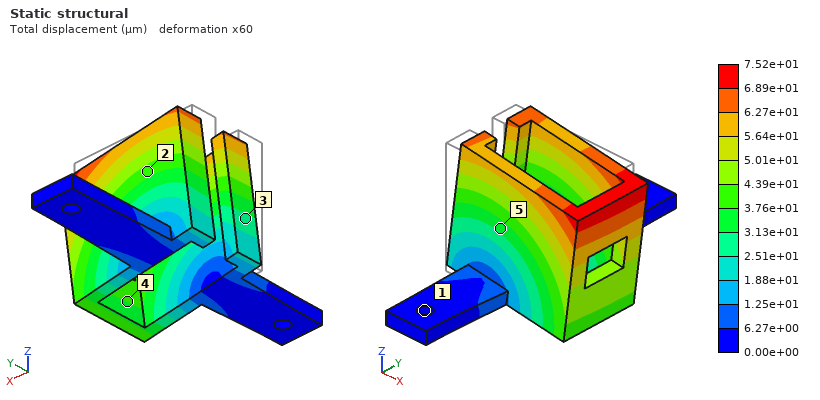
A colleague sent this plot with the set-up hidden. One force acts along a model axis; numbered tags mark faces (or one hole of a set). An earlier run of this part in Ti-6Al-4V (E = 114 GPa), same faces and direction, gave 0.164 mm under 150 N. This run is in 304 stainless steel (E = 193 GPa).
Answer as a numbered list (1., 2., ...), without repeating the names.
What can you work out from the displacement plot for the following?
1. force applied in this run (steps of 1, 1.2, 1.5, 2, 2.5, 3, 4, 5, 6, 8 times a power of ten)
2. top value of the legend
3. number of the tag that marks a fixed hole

1. 120 N
2. 7.52e+01 µm
3. 1
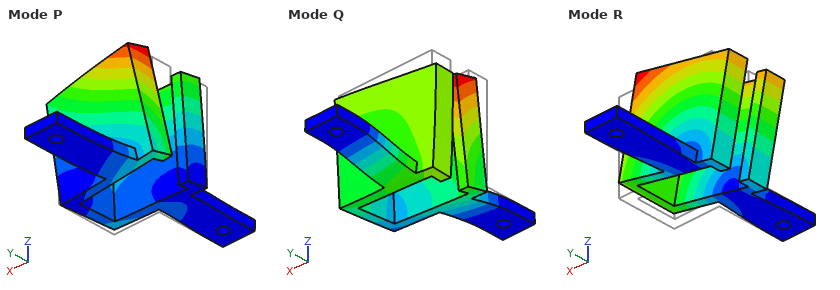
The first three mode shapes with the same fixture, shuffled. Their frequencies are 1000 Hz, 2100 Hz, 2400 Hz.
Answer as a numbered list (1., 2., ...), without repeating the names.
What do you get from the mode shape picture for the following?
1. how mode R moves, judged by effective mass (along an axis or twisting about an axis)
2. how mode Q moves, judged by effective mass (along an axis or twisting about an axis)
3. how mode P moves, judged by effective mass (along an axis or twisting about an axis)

1. along X
2. along Z
3. along Y
